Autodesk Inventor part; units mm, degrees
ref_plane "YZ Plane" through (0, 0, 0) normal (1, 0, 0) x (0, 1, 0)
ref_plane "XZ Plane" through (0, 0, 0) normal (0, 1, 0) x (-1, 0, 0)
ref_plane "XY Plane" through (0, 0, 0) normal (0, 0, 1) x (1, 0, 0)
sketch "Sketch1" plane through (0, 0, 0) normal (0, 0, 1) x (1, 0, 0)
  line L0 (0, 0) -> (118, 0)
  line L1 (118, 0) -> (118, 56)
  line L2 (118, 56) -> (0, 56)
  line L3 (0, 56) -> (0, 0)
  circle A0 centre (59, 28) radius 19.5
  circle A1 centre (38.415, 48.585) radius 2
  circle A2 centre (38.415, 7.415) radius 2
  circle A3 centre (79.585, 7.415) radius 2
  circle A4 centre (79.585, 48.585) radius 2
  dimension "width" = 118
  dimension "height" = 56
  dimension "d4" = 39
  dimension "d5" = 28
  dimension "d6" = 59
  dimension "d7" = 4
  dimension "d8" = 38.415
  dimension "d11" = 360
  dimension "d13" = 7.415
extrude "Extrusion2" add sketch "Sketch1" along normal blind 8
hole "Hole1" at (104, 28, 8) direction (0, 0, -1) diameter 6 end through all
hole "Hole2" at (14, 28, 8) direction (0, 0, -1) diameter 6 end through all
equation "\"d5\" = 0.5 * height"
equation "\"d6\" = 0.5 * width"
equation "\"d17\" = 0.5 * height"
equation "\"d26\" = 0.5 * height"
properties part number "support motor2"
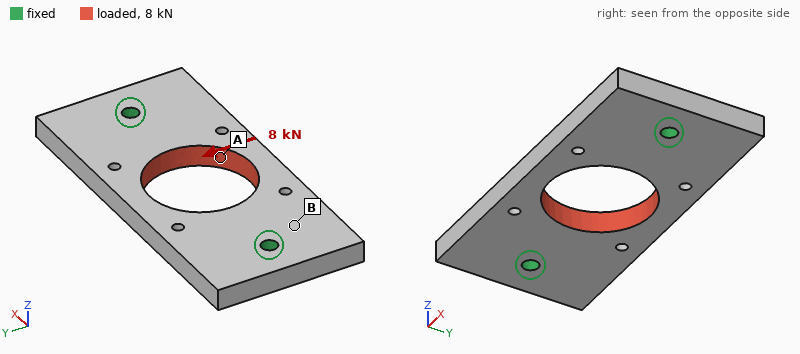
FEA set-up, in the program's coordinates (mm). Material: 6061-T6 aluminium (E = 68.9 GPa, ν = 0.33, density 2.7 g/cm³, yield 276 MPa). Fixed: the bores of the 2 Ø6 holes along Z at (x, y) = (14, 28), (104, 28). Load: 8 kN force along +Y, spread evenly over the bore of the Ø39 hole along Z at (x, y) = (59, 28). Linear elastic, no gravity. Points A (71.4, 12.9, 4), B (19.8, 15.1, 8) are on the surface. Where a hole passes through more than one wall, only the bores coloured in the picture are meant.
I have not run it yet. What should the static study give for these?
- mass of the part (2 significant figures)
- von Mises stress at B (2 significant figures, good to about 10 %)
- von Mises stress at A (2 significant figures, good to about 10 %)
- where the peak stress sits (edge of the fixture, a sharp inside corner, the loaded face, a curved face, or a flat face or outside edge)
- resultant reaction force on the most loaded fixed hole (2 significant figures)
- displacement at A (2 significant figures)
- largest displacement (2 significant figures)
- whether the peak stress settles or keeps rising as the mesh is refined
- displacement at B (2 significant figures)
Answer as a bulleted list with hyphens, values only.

- 110 g
- 15 MPa
- 32 MPa
- edge of the fixture
- 4.0 kN
- 29 µm
- 34 µm
- keeps rising
- 8.2 µm
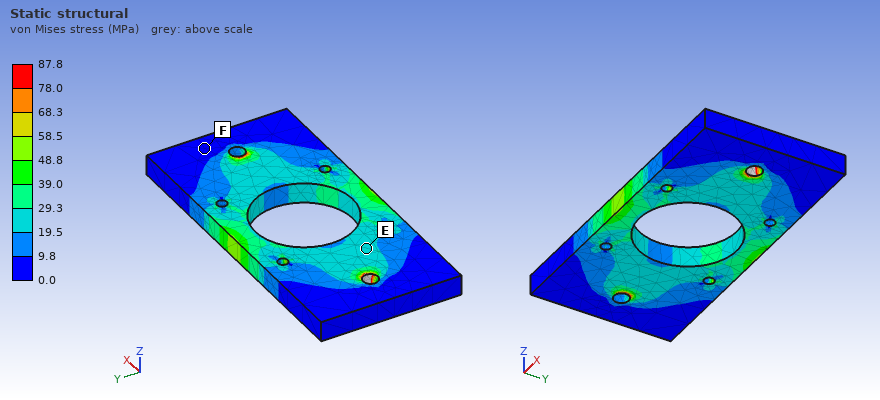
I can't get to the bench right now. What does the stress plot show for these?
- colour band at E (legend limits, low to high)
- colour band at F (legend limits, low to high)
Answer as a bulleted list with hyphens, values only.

- 19.5 to 29.3 MPa
- 0.0 to 9.8 MPa
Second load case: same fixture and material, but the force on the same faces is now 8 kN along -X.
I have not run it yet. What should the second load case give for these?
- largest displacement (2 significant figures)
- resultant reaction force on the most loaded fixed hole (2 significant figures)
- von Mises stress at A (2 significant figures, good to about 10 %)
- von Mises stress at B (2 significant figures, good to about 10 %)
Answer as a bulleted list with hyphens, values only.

- 12 µm
- 4.0 kN
- 19 MPa
- 9.1 MPa
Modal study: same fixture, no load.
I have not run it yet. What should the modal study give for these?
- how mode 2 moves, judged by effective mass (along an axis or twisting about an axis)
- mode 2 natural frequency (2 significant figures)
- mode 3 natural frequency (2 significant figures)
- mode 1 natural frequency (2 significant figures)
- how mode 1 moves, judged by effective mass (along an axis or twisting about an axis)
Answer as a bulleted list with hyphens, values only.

- along Z
- 4400 Hz
- 6800 Hz
- 4200 Hz
- twisting about X
